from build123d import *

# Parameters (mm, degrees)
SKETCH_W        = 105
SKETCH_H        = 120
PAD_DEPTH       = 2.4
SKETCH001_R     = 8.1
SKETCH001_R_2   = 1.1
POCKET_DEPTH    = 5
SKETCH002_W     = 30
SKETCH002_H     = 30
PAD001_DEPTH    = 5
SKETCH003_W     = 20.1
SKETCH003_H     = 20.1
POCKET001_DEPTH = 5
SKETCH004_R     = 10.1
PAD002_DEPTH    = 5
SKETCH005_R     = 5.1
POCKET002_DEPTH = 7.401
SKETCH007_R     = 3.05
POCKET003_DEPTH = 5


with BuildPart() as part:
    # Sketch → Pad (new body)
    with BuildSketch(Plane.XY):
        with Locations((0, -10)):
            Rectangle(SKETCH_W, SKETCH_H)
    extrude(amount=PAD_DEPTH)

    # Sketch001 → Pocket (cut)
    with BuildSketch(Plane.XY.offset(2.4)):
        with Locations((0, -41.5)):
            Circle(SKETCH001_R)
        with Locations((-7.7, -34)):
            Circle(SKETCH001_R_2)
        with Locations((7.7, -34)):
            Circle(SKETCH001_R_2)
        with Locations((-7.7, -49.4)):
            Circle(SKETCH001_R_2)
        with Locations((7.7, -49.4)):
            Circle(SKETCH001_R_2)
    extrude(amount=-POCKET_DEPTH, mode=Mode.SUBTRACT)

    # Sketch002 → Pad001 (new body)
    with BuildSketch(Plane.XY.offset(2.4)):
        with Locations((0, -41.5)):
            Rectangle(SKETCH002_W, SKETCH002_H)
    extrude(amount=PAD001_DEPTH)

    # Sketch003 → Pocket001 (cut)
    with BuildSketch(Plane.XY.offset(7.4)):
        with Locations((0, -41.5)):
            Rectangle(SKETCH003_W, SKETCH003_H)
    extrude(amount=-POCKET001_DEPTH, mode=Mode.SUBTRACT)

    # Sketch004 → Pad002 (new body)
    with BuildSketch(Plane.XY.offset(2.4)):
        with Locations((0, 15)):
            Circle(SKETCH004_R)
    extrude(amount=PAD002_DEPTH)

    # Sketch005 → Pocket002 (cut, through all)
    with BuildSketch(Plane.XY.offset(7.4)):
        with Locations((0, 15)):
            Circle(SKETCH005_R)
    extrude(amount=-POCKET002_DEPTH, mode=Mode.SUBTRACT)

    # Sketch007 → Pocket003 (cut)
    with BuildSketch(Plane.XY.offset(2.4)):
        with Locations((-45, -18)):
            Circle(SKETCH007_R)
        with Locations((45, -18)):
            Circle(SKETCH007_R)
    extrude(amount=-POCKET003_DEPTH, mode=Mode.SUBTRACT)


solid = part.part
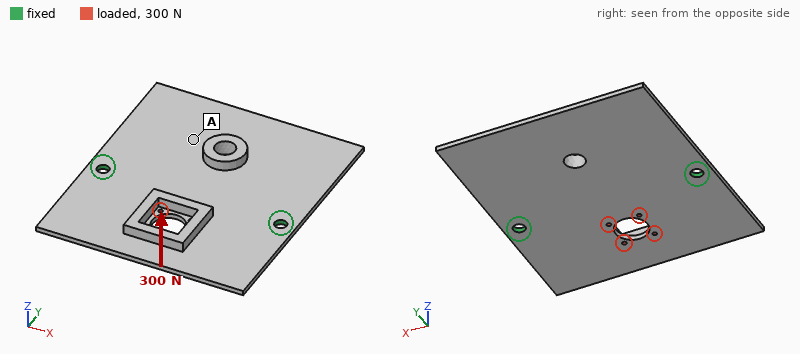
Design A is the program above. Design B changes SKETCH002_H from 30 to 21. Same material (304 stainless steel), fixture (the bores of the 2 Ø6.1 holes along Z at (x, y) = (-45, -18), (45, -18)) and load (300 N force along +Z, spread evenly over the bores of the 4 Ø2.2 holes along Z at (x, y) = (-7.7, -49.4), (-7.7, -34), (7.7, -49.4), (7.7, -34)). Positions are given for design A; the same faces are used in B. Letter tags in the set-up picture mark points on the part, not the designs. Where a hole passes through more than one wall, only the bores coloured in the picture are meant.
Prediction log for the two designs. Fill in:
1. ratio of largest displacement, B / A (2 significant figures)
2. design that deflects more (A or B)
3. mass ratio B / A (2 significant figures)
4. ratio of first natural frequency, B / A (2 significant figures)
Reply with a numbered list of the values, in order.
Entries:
1. 1.2
2. B
3. 0.96
4. 1.00
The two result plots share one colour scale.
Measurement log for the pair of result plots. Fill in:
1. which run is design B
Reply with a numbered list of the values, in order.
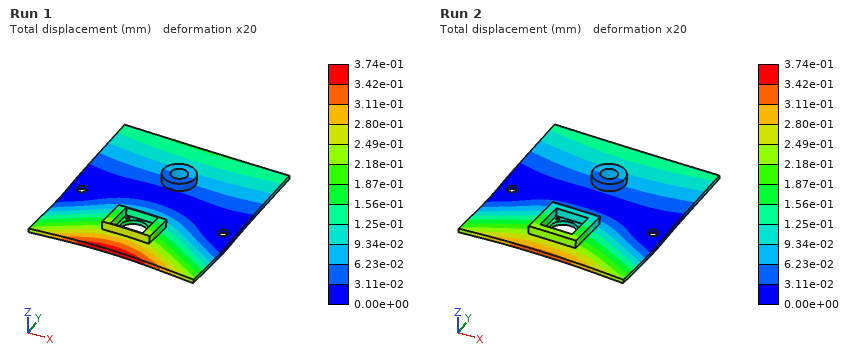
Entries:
1. Run 1
